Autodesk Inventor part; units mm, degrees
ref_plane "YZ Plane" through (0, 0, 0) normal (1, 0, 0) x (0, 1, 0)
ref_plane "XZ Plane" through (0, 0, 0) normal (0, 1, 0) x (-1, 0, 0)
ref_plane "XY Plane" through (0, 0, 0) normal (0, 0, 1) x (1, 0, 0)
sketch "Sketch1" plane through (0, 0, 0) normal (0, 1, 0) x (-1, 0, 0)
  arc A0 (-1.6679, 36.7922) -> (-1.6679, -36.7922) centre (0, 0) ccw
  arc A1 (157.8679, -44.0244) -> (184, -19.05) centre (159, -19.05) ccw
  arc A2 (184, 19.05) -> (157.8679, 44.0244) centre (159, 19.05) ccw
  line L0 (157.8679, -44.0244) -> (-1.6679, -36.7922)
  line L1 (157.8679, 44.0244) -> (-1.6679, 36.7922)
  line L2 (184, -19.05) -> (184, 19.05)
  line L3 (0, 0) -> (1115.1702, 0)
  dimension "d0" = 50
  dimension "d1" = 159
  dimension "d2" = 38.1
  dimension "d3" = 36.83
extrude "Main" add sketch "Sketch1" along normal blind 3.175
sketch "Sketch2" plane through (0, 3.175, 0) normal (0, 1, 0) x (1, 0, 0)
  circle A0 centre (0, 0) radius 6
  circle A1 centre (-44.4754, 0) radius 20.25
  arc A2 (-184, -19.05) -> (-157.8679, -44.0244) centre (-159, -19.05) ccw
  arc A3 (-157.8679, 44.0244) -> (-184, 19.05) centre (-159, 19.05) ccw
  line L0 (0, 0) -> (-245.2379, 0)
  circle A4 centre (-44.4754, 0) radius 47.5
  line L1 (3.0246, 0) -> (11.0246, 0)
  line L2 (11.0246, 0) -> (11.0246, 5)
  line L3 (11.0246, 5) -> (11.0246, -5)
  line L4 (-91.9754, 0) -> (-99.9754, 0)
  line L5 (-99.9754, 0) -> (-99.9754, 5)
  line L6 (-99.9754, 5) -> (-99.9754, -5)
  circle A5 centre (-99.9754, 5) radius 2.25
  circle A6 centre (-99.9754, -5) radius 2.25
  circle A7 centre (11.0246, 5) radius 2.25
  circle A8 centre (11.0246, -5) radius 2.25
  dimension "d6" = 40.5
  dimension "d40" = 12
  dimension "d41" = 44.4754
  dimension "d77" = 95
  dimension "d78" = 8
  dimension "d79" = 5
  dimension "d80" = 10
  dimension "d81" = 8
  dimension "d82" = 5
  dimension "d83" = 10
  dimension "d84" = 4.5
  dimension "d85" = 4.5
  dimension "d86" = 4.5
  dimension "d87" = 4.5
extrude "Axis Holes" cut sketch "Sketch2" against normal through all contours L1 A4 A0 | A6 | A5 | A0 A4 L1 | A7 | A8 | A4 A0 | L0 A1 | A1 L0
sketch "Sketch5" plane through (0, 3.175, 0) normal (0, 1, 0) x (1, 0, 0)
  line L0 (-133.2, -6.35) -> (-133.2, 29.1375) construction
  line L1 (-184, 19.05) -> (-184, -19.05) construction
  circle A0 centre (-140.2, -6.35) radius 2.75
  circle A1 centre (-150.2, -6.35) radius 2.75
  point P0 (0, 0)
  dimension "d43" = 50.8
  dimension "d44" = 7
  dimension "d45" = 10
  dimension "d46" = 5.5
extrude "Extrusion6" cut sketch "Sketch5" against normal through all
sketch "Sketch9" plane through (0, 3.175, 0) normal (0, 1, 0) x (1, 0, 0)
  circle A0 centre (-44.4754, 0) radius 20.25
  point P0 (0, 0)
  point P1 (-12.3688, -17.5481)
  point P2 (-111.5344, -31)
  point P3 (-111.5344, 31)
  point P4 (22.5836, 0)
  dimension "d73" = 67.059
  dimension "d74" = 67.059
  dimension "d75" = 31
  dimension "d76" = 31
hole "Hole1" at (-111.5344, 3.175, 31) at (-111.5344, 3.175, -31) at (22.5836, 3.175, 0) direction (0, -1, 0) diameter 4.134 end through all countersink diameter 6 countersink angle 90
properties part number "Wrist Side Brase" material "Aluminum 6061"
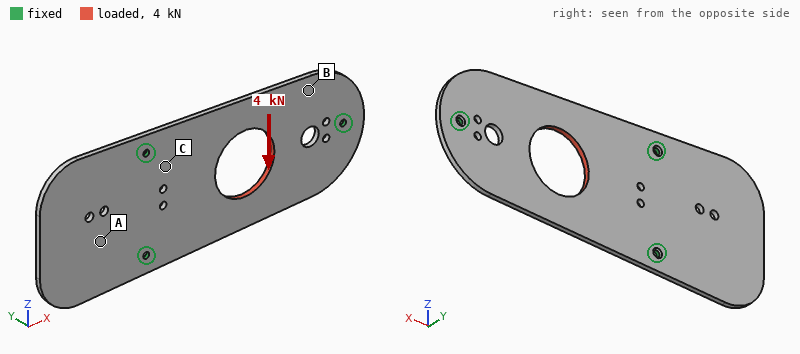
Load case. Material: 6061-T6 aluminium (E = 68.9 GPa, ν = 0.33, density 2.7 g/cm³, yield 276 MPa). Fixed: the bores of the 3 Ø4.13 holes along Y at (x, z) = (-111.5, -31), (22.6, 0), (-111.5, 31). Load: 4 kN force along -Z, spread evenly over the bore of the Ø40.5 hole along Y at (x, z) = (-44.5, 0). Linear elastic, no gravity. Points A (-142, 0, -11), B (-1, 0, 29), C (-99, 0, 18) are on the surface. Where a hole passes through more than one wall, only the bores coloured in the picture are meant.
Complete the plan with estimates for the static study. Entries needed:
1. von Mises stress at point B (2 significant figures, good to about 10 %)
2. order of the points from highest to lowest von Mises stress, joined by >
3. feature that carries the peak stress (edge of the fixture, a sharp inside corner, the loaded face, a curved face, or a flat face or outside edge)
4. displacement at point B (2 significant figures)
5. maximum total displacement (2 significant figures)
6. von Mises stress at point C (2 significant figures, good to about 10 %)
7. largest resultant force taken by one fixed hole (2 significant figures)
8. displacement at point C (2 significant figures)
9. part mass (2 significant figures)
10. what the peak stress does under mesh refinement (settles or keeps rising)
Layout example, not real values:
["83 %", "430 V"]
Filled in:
["15 MPa", "C > B > A", "edge of the fixture", "28 µm", "46 µm", "24 MPa", "1.6 kN", "9.3 µm", "130 g", "keeps rising"]
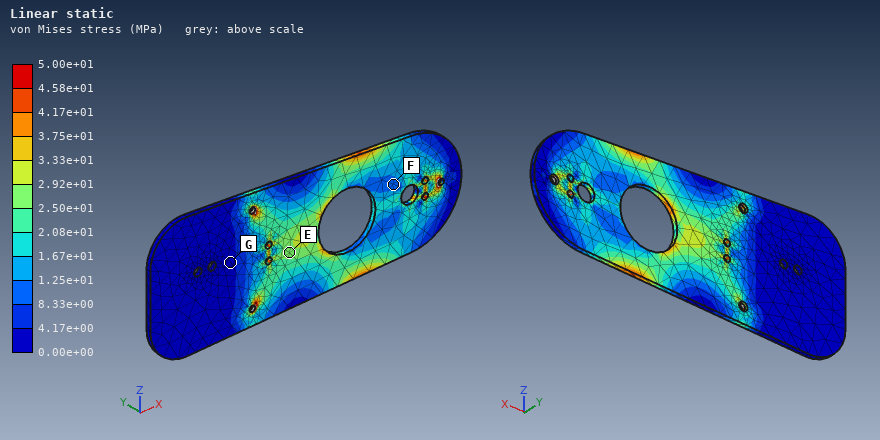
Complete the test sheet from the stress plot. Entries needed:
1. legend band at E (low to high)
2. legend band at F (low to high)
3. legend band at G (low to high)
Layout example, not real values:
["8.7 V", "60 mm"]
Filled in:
["2.50e+01 to 2.92e+01 MPa", "8.33e+00 to 1.25e+01 MPa", "0.00e+00 to 4.17e+00 MPa"]
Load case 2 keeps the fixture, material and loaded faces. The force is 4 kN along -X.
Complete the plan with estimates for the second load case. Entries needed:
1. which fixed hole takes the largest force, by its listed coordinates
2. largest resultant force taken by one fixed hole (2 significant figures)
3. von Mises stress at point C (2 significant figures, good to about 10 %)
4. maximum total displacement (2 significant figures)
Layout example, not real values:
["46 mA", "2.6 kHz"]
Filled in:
["(22.6, 0)", "1.5 kN", "11 MPa", "15 µm"]
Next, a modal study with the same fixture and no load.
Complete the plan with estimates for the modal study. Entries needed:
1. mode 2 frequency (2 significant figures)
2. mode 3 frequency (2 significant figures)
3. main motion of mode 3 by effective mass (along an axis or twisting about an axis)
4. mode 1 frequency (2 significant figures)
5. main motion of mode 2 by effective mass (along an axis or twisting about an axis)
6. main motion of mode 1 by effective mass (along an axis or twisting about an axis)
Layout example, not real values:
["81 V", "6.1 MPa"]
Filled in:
["790 Hz", "970 Hz", "twisting about X", "460 Hz", "along Y", "along Y"]
